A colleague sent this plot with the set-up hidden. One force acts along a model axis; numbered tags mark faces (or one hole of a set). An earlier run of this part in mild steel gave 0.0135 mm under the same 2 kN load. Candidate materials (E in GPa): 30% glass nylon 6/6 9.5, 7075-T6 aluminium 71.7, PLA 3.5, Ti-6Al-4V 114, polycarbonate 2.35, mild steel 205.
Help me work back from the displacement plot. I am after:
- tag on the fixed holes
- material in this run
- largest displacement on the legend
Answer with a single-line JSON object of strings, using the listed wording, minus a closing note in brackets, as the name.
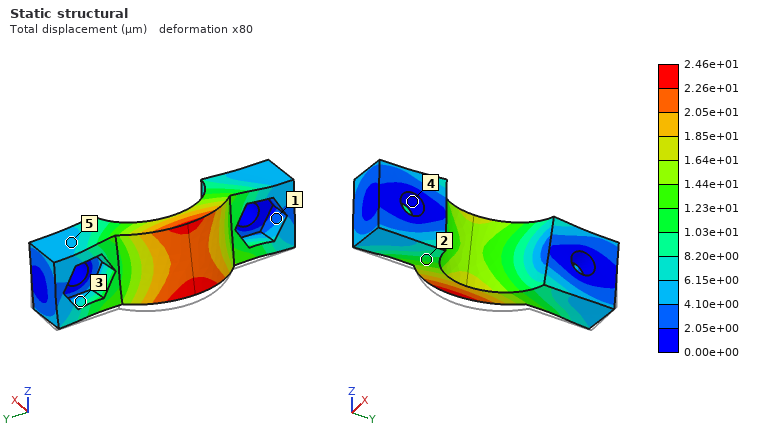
{"tag on the fixed holes": "4", "material in this run": "Ti-6Al-4V", "largest displacement on the legend": "2.46e+01 µm"}
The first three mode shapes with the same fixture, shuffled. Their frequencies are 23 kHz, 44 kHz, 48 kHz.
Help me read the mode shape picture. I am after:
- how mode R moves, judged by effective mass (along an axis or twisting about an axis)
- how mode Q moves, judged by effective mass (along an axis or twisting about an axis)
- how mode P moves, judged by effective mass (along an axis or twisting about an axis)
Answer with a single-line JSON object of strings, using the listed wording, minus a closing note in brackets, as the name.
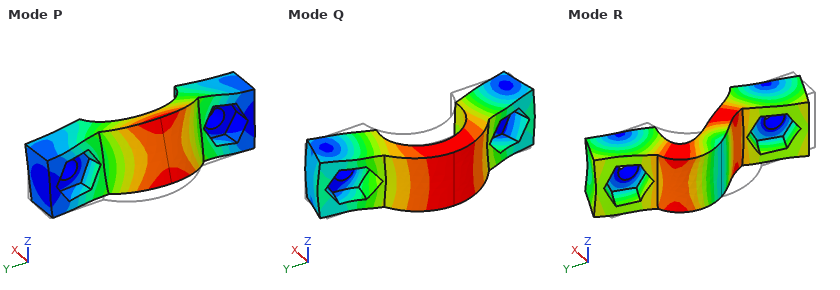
{"how mode R moves, judged by effective mass": "along Y", "how mode Q moves, judged by effective mass": "along X", "how mode P moves, judged by effective mass": "along Z"}
